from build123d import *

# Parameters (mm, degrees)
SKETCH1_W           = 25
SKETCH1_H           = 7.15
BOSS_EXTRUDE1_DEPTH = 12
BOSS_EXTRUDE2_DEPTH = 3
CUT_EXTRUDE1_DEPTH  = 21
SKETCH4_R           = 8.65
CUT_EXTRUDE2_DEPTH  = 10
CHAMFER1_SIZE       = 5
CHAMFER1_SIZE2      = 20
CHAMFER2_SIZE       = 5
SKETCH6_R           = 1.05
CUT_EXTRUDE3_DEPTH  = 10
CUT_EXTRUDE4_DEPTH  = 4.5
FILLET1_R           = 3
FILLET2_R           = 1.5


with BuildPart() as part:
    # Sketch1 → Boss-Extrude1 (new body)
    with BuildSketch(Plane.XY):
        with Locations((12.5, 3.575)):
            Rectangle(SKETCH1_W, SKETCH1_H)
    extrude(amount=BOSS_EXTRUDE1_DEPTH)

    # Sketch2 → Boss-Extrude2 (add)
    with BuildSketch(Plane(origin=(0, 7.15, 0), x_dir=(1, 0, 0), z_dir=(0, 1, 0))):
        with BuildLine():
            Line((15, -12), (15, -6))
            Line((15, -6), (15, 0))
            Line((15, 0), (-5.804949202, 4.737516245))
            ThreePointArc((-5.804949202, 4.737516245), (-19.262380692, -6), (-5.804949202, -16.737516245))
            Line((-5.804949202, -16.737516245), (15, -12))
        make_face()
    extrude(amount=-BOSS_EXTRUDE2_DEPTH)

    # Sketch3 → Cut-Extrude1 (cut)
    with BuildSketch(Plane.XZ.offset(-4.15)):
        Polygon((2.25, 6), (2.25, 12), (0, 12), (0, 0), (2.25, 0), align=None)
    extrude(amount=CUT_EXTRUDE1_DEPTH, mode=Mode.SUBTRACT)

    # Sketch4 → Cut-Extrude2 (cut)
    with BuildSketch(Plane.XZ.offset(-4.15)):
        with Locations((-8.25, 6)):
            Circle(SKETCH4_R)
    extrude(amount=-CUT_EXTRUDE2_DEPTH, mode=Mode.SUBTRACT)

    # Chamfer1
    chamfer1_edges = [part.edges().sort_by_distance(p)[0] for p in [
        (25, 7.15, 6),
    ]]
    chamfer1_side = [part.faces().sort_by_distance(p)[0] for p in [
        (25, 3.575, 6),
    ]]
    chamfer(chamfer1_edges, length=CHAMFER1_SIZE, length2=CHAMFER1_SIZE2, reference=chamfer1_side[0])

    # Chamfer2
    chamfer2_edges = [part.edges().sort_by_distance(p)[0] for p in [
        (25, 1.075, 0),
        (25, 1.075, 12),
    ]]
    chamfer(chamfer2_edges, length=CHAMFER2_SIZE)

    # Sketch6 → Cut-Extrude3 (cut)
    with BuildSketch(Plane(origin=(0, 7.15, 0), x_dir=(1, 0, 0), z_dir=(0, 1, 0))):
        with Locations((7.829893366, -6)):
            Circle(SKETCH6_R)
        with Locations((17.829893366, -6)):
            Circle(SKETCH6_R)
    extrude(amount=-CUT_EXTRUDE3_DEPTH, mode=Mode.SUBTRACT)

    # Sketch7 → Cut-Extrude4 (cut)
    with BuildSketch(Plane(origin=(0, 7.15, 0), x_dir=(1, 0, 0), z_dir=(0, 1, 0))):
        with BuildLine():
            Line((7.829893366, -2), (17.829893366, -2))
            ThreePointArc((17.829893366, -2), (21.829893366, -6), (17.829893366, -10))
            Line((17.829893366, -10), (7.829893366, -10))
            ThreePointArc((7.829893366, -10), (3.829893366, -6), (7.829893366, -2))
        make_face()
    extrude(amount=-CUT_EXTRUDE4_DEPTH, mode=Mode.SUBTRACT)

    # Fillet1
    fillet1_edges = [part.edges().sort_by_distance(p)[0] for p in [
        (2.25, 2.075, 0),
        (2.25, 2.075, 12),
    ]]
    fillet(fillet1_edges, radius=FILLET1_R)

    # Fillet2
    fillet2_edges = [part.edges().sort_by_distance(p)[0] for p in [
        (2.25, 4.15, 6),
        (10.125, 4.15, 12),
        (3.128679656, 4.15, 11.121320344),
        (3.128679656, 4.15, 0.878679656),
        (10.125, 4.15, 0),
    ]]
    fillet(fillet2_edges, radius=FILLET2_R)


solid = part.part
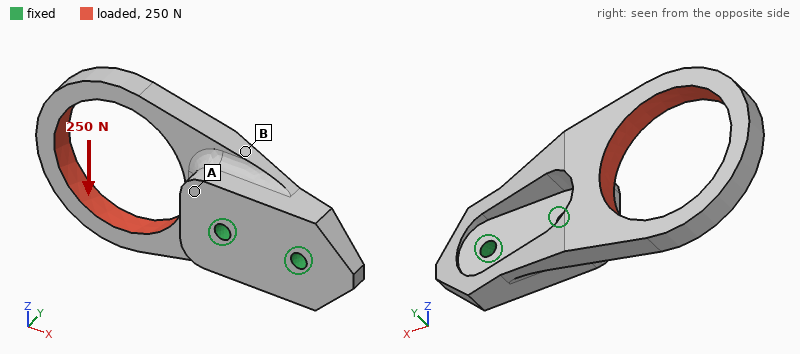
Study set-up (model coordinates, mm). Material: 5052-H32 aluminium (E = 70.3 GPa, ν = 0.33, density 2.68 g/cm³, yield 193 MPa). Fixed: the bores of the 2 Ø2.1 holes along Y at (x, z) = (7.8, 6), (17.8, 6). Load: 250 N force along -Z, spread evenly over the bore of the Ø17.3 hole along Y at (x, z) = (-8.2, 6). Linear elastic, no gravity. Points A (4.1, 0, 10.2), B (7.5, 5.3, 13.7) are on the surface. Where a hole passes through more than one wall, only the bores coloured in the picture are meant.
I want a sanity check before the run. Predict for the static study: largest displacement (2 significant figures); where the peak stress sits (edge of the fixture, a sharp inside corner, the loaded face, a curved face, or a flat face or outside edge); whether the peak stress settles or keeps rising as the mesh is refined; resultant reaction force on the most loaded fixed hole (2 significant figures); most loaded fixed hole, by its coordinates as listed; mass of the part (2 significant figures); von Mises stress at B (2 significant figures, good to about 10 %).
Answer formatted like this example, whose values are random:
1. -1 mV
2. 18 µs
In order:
1. 0.12 mm
2. edge of the fixture
3. keeps rising
4. 570 N
5. (7.8, 6)
6. 4.1 g
7. 31 MPa
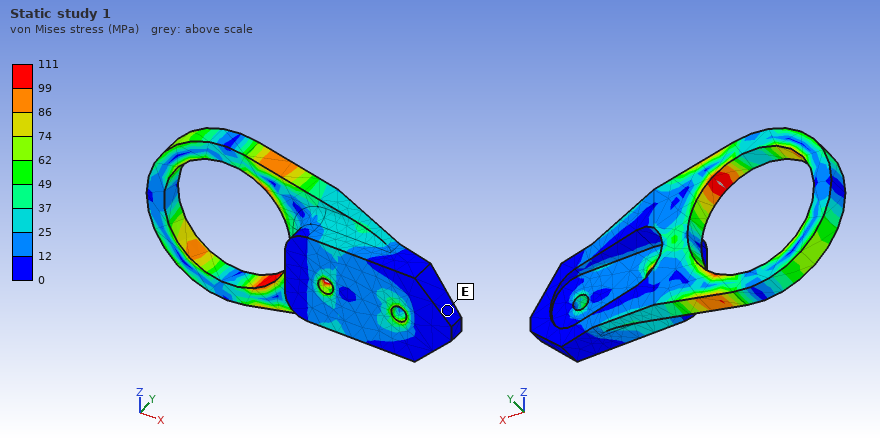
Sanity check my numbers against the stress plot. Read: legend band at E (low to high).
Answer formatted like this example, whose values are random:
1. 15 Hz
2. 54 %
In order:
1. 0 to 12 MPa
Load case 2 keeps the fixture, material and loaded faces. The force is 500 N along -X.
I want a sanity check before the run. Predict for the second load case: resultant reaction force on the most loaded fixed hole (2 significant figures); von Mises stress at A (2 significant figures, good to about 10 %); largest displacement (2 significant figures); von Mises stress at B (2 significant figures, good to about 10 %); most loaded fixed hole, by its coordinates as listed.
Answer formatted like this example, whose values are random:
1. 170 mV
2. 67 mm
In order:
1. 320 N
2. 7.1 MPa
3. 48 µm
4. 37 MPa
5. (17.8, 6)
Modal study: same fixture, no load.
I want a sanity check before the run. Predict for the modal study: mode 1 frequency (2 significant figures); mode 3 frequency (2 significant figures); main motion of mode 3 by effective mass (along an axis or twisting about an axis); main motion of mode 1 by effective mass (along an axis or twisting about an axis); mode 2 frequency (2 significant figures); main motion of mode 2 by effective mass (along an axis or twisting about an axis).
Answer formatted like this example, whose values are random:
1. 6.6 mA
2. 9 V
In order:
1. 4000 Hz
2. 8000 Hz
3. twisting about X
4. along Y
5. 7300 Hz
6. along Z
